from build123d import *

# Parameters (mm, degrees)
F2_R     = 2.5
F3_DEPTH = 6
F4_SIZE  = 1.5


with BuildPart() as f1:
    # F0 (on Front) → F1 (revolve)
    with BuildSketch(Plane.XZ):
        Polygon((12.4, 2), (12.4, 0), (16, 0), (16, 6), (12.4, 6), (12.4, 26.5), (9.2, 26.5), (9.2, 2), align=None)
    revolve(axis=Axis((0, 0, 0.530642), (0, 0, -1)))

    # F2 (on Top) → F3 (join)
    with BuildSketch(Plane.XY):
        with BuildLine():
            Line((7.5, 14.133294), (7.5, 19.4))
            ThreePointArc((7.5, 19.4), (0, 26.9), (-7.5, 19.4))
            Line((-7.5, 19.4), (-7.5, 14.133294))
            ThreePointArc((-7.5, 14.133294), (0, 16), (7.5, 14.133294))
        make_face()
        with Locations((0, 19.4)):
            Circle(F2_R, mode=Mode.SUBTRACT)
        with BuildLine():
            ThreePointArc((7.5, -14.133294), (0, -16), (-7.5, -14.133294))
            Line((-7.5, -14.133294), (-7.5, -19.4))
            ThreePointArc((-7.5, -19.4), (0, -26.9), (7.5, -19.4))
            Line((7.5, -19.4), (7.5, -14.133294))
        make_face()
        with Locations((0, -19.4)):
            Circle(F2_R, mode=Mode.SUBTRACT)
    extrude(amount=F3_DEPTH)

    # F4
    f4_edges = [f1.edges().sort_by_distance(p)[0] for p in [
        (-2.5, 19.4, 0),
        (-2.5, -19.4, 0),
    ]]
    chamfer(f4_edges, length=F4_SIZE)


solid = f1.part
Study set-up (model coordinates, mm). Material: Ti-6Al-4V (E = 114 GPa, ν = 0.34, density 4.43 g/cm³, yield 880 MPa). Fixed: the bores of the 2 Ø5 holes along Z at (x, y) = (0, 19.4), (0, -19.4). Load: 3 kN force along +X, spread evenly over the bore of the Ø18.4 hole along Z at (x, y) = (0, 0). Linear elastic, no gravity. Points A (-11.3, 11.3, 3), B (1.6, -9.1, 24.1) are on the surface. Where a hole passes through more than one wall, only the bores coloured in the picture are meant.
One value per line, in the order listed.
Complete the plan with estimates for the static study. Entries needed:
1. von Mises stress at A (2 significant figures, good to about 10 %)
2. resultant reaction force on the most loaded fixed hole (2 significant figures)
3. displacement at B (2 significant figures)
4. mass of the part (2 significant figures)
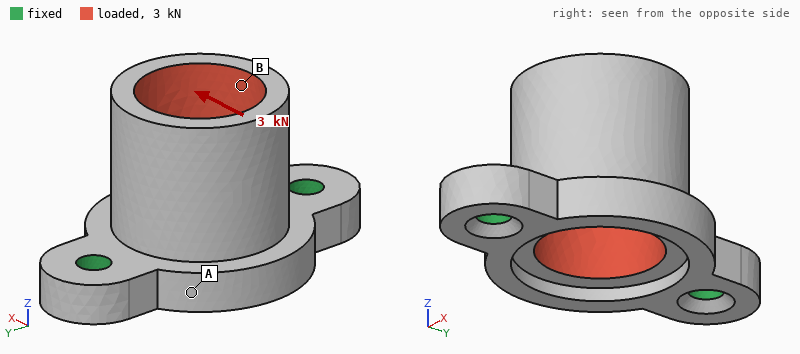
70 MPa
1.5 kN
0.10 mm
39 g
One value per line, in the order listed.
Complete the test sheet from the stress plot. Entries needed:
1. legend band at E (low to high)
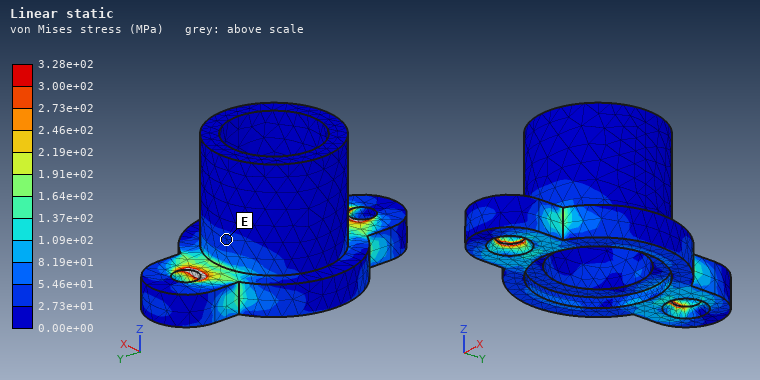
2.73e+01 to 5.46e+01 MPa
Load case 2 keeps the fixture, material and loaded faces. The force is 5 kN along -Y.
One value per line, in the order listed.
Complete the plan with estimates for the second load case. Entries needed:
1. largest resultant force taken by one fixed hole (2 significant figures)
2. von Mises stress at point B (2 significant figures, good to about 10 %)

3.1 kN
17 MPa
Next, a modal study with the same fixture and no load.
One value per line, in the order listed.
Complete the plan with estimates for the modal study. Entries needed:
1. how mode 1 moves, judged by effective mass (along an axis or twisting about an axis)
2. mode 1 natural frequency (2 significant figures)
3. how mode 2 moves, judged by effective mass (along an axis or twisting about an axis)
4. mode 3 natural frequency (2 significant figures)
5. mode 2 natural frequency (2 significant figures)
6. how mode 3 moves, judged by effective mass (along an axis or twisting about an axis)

along X
5300 Hz
along Z
14 kHz
13 kHz
along Y
